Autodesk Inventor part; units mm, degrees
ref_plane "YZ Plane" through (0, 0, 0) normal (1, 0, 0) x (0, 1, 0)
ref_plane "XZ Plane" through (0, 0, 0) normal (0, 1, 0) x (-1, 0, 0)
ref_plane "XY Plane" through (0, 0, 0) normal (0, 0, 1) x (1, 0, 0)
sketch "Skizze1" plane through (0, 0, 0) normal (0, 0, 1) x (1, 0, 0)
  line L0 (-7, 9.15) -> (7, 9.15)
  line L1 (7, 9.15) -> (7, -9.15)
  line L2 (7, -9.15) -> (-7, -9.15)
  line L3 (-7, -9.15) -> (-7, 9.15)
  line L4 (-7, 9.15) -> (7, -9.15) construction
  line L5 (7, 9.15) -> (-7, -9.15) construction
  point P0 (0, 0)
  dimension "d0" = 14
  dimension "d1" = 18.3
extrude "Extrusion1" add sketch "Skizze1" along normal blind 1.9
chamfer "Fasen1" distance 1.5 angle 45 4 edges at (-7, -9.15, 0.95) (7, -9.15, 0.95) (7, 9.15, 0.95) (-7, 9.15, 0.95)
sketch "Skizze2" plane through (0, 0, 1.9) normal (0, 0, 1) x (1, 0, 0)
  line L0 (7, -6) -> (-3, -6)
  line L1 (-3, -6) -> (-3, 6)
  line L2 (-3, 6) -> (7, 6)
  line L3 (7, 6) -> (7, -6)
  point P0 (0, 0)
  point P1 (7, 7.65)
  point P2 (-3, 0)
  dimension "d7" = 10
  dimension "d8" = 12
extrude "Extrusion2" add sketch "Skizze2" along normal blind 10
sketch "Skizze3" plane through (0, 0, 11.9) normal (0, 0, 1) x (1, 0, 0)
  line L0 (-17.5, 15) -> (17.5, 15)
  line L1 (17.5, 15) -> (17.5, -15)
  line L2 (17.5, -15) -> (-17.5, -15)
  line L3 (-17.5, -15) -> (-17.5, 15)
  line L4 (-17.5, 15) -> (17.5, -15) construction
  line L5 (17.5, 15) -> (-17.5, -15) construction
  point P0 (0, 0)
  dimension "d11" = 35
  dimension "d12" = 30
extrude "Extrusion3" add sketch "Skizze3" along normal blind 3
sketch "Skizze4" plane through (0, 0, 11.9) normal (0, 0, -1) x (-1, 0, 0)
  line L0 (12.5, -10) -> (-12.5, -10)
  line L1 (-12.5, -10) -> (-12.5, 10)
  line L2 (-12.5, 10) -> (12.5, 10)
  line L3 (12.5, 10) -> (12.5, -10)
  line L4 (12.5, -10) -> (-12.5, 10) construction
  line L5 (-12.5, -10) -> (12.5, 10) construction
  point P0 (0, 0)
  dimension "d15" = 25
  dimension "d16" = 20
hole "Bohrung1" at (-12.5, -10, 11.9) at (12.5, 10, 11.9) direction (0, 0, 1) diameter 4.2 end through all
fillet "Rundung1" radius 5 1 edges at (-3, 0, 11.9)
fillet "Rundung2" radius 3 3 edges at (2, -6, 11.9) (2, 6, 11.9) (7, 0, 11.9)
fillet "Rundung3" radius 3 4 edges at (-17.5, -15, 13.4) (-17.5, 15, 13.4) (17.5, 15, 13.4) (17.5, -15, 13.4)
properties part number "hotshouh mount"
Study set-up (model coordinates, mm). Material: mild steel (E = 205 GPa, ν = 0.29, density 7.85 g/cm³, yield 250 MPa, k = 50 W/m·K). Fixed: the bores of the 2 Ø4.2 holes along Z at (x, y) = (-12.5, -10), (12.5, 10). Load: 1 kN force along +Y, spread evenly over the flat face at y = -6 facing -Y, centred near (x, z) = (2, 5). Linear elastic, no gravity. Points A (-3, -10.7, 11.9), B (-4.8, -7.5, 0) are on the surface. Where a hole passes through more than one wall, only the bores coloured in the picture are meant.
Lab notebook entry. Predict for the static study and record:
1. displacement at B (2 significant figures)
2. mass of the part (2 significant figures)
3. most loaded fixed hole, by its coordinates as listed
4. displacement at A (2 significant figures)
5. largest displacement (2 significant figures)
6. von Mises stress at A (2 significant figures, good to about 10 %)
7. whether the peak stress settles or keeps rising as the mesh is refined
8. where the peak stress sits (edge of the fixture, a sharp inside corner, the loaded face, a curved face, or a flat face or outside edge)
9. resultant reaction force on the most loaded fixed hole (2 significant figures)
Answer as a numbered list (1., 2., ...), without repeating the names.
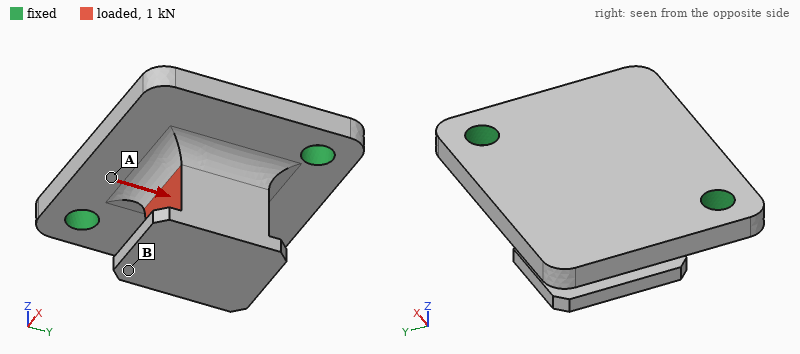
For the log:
1. 27 µm
2. 38 g
3. (12.5, 10)
4. 11 µm
5. 38 µm
6. 45 MPa
7. keeps rising
8. edge of the fixture
9. 600 N
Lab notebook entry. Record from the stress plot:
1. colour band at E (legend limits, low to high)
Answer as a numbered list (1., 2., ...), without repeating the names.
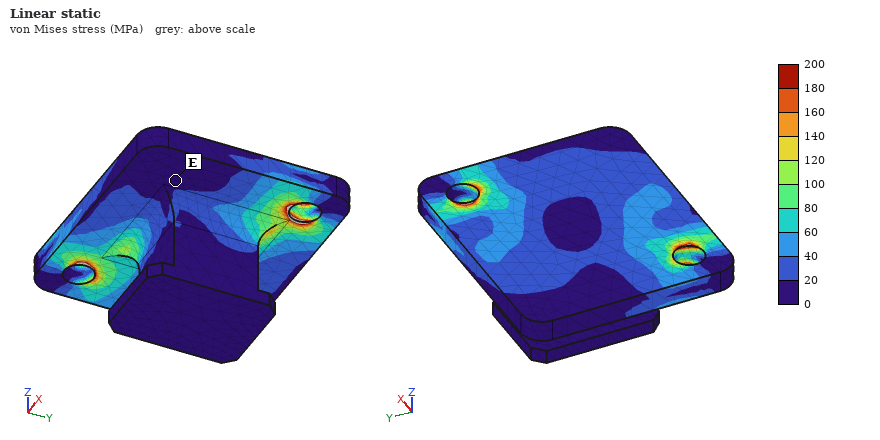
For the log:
1. 0 to 20 MPa
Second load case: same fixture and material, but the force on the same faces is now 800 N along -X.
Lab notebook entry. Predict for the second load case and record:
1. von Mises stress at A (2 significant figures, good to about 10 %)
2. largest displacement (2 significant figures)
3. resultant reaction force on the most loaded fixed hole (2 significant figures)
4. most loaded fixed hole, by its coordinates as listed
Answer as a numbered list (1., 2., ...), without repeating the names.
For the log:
1. 33 MPa
2. 25 µm
3. 530 N
4. (-12.5, -10)
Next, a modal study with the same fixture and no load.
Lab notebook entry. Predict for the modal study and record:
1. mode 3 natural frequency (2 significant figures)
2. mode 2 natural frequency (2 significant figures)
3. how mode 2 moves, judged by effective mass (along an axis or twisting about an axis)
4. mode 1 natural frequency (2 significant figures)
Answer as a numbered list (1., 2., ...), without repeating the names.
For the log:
1. 17 kHz
2. 10 kHz
3. along Z
4. 5300 Hz
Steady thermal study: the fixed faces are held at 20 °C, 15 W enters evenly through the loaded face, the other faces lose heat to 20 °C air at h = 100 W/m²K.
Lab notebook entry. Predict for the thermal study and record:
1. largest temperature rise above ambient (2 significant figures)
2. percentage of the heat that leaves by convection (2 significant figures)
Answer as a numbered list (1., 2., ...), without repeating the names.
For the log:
1. 46 K
2. 36 %
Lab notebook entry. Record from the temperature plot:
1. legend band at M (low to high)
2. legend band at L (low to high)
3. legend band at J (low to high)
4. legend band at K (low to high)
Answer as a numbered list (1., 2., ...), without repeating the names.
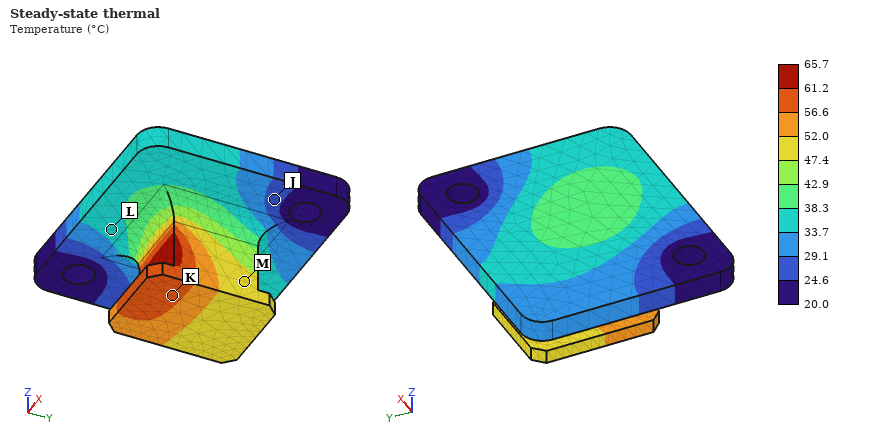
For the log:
1. 47.4 to 52.0 °C
2. 33.7 to 38.3 °C
3. 24.6 to 29.1 °C
4. 56.6 to 61.2 °C
